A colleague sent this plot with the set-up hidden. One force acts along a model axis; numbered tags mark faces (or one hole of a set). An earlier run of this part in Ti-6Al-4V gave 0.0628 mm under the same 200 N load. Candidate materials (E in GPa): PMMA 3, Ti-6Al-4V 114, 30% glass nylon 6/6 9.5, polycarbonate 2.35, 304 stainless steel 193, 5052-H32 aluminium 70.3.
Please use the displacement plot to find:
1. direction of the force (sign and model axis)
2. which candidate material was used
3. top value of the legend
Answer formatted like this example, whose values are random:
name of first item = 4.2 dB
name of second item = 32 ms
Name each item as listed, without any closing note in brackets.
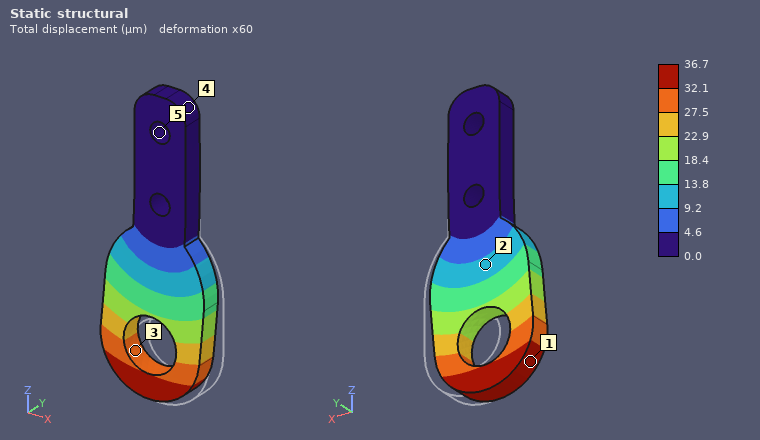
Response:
direction of the force = -X
which candidate material was used = 304 stainless steel
top value of the legend = 36.7 µm
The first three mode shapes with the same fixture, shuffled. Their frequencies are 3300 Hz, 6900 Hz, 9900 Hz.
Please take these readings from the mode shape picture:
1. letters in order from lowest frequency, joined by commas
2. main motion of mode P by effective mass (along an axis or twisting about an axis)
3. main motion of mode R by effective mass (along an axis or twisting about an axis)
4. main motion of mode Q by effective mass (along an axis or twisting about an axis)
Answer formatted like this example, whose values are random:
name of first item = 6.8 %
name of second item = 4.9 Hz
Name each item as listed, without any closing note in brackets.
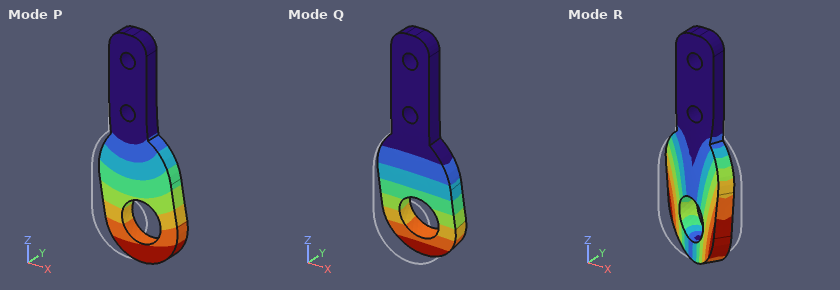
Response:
letters in order from lowest frequency, joined by commas = Q, P, R
main motion of mode P by effective mass = along X
main motion of mode R by effective mass = twisting about Z
main motion of mode Q by effective mass = along Y
